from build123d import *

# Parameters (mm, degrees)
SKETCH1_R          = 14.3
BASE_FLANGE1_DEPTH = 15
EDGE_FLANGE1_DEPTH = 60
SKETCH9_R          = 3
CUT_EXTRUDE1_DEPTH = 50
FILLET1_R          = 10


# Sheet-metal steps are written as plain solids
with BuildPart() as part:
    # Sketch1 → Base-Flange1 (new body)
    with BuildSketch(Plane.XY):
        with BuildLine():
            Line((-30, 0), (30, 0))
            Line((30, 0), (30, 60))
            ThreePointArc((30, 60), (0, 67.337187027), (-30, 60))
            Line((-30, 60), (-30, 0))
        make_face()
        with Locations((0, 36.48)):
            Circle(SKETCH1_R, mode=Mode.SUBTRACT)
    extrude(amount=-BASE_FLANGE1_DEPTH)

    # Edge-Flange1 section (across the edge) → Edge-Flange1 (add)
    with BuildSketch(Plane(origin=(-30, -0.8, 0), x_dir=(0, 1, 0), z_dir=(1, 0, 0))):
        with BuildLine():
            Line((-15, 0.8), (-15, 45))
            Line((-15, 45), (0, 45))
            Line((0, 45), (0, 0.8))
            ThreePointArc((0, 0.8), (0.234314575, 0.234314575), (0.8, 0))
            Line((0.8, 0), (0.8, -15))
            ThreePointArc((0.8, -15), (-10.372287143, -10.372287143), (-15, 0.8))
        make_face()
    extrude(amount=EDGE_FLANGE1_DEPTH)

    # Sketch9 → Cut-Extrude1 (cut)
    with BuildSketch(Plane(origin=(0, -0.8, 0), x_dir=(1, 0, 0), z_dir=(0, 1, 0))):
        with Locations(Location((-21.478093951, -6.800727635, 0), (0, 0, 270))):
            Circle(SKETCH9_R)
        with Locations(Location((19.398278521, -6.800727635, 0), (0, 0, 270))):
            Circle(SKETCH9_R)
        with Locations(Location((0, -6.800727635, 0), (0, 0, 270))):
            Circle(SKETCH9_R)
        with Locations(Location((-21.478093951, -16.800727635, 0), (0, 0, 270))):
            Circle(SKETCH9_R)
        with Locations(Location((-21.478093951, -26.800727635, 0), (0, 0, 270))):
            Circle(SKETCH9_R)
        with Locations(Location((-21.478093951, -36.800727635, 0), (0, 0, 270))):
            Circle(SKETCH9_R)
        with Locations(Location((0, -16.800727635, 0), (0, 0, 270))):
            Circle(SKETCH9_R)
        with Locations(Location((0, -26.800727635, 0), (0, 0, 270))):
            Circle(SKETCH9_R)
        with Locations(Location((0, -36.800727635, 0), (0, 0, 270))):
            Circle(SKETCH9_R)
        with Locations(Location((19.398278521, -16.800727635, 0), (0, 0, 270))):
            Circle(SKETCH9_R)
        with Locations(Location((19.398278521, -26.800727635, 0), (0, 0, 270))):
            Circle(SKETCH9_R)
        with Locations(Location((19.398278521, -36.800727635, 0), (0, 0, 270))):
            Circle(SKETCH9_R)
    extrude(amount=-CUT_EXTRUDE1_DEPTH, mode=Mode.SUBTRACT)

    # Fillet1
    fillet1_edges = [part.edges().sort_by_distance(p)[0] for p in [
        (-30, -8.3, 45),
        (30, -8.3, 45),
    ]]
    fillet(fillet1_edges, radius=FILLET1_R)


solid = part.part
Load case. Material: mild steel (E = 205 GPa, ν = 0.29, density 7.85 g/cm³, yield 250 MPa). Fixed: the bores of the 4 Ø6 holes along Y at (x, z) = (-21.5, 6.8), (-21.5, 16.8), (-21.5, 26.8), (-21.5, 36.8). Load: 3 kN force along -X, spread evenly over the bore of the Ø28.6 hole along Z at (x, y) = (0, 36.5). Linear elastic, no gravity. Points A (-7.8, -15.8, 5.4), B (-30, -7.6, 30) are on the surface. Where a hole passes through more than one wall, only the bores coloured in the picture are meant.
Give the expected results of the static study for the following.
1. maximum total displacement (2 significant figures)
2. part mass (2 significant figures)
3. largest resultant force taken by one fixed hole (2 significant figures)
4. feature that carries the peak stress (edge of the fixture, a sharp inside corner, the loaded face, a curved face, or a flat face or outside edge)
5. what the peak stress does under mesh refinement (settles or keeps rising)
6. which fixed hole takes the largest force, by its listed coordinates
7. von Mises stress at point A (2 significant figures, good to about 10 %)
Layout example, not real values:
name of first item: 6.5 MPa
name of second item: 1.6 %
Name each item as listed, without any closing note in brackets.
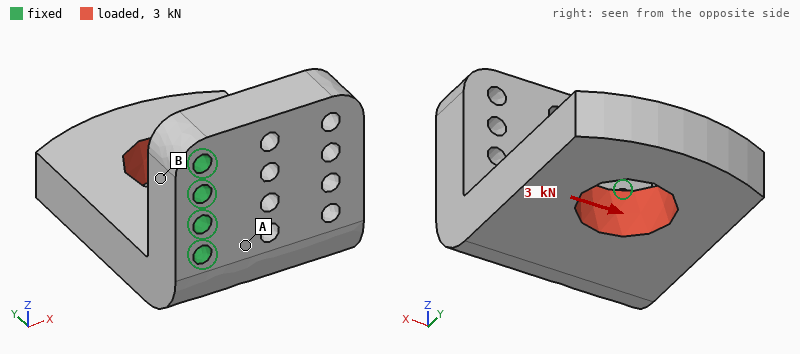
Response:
maximum total displacement: 76 µm
part mass: 740 g
largest resultant force taken by one fixed hole: 4.0 kN
feature that carries the peak stress: edge of the fixture
what the peak stress does under mesh refinement: keeps rising
which fixed hole takes the largest force, by its listed coordinates: (-21.5, 6.8)
von Mises stress at point A: 44 MPa
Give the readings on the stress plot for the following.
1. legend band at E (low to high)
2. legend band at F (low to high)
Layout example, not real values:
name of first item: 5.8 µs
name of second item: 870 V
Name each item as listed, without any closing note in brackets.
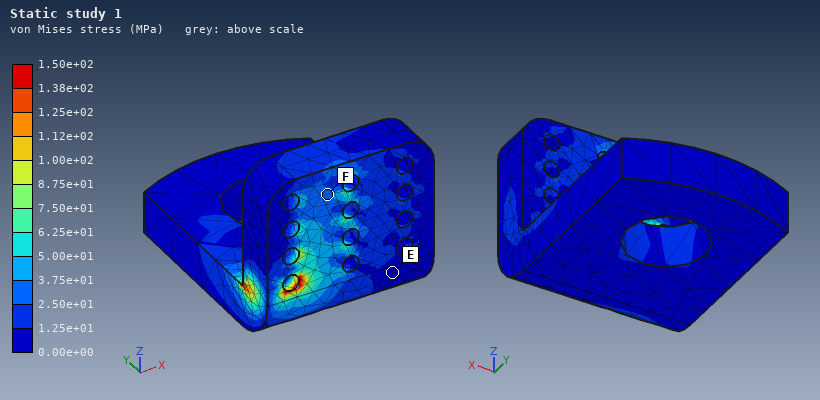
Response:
legend band at E: 0.00e+00 to 1.25e+01 MPa
legend band at F: 2.50e+01 to 3.75e+01 MPa
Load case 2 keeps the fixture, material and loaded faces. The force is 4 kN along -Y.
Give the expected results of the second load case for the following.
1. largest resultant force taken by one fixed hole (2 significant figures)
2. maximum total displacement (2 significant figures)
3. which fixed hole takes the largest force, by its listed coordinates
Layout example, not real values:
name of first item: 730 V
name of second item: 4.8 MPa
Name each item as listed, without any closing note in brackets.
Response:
largest resultant force taken by one fixed hole: 3.8 kN
maximum total displacement: 54 µm
which fixed hole takes the largest force, by its listed coordinates: (-21.5, 6.8)
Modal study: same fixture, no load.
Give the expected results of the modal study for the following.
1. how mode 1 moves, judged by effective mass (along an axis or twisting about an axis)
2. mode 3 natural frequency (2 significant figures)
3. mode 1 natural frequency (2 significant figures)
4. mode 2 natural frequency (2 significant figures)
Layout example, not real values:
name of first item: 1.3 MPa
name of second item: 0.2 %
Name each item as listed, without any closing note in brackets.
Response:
how mode 1 moves, judged by effective mass: along Z
mode 3 natural frequency: 4500 Hz
mode 1 natural frequency: 1500 Hz
mode 2 natural frequency: 1900 Hz
